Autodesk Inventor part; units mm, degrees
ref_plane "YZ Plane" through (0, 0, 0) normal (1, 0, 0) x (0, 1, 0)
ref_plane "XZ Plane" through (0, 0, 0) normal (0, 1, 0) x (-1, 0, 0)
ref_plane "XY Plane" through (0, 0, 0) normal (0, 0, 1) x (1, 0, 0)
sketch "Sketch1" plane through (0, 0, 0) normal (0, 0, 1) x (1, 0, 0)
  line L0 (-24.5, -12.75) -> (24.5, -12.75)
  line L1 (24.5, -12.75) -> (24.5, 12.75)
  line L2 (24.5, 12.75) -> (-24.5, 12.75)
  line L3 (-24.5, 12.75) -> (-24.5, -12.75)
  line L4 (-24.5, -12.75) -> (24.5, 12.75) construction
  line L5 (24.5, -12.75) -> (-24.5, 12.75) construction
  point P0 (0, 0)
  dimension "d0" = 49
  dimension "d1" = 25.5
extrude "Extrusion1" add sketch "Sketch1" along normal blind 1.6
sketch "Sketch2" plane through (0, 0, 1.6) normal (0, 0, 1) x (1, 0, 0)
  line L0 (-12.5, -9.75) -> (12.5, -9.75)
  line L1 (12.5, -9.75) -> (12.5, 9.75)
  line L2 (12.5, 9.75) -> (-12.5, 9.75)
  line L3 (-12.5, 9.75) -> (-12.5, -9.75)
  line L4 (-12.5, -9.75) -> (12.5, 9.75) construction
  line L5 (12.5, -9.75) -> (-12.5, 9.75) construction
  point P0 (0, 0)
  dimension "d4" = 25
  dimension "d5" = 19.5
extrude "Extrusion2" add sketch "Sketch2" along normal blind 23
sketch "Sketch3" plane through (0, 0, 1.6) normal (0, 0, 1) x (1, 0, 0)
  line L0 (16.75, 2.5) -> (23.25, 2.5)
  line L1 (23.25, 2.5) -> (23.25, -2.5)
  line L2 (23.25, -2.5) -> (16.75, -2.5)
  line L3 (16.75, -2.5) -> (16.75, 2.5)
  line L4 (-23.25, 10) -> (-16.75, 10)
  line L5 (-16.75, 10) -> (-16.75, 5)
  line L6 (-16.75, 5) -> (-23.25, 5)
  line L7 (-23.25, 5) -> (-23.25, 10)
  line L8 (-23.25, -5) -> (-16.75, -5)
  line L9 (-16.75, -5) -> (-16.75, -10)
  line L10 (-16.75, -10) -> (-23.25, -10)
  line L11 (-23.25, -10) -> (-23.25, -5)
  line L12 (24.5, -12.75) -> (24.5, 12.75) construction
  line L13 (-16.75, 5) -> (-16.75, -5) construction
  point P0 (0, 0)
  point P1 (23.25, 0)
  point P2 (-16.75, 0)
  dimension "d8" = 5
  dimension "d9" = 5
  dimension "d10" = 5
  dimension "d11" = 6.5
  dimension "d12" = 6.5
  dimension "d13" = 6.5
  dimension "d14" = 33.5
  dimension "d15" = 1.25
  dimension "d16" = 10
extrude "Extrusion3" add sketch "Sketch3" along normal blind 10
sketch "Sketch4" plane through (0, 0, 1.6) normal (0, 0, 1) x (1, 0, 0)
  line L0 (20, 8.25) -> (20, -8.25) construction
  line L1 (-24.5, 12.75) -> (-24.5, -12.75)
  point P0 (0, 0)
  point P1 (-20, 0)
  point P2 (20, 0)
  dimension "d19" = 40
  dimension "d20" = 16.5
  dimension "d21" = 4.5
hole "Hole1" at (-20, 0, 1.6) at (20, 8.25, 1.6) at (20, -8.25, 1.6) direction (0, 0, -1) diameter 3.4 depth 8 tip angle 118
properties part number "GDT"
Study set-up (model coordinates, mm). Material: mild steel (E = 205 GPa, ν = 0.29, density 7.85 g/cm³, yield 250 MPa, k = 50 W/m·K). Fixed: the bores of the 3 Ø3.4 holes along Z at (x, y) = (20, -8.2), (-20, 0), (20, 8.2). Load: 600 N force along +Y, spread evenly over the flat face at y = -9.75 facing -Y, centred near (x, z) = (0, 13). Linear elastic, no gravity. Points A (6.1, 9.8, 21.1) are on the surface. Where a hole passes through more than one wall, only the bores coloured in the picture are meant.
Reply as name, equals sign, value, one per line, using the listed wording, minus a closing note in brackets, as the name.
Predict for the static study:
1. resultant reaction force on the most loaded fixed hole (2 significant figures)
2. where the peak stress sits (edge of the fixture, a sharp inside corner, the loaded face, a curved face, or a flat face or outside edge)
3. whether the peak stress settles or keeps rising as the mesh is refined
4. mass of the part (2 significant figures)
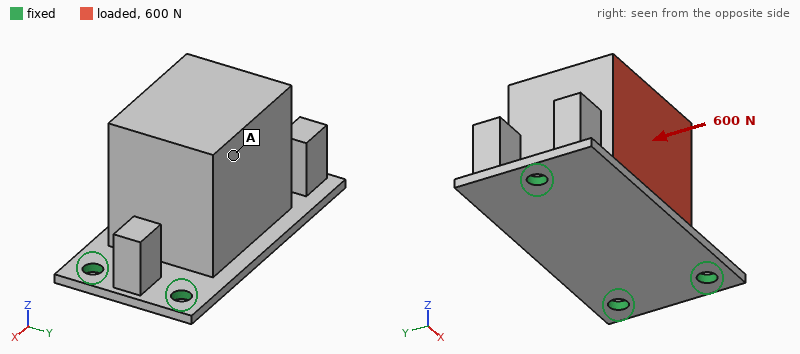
resultant reaction force on the most loaded fixed hole = 490 N
where the peak stress sits = edge of the fixture
whether the peak stress settles or keeps rising as the mesh is refined = keeps rising
mass of the part = 110 g
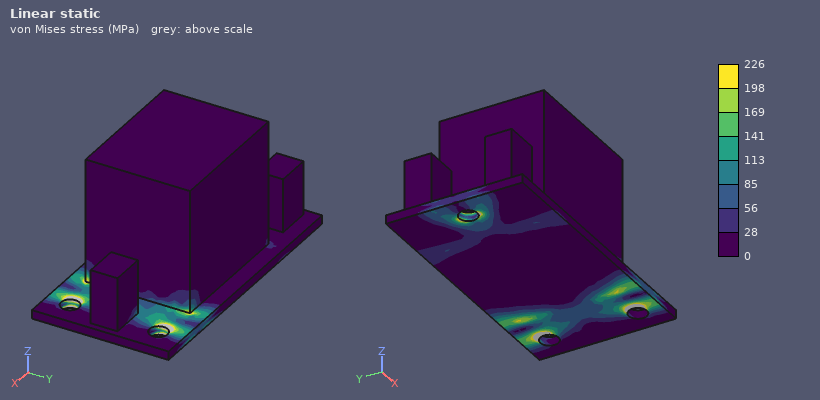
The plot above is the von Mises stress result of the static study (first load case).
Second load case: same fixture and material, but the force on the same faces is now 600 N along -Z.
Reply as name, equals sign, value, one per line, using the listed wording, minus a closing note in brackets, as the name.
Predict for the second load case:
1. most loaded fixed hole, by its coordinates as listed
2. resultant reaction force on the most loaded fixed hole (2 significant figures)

most loaded fixed hole, by its coordinates as listed = (20, -8.2)
resultant reaction force on the most loaded fixed hole = 480 N
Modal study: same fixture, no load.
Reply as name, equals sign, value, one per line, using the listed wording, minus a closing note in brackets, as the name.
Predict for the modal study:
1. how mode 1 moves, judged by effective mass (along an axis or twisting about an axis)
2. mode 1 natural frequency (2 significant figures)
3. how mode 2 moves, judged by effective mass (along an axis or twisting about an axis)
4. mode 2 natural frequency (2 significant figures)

how mode 1 moves, judged by effective mass = along Y
mode 1 natural frequency = 1900 Hz
how mode 2 moves, judged by effective mass = along Z
mode 2 natural frequency = 3500 Hz
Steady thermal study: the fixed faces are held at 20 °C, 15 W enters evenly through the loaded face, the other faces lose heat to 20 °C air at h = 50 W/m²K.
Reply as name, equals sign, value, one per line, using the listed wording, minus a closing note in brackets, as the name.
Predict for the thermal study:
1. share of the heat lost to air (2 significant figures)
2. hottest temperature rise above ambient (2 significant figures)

share of the heat lost to air = 35 %
hottest temperature rise above ambient = 37 K
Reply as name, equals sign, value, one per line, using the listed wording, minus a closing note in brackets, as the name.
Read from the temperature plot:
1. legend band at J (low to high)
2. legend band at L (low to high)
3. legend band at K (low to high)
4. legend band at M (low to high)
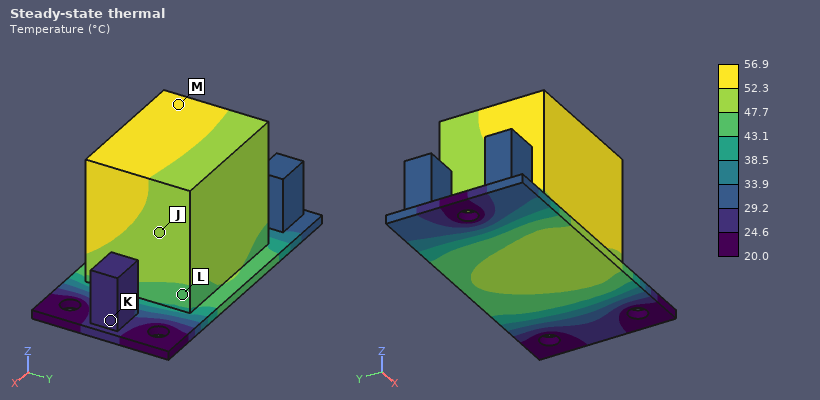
legend band at J = 47.7 to 52.3 °C
legend band at L = 43.1 to 47.7 °C
legend band at K = 24.6 to 29.2 °C
legend band at M = 52.3 to 56.9 °C
